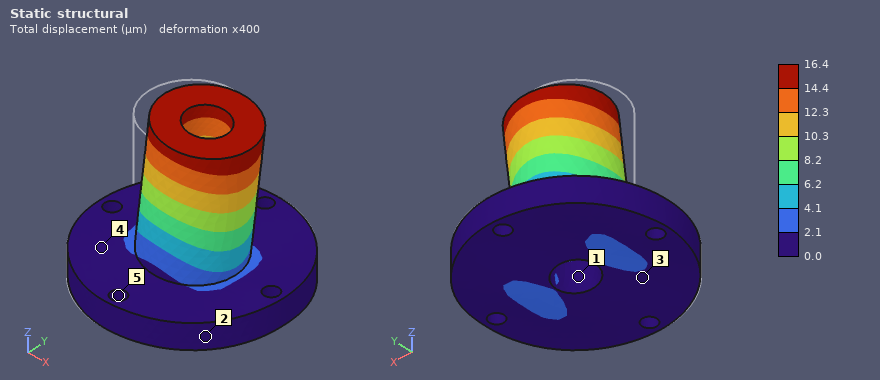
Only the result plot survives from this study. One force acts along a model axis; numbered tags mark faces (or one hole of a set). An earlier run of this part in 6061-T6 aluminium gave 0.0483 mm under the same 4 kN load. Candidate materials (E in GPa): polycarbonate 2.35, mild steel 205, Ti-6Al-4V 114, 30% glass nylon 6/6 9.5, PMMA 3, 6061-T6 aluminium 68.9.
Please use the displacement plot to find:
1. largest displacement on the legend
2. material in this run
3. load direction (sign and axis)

16.4 µm
mild steel
+X
